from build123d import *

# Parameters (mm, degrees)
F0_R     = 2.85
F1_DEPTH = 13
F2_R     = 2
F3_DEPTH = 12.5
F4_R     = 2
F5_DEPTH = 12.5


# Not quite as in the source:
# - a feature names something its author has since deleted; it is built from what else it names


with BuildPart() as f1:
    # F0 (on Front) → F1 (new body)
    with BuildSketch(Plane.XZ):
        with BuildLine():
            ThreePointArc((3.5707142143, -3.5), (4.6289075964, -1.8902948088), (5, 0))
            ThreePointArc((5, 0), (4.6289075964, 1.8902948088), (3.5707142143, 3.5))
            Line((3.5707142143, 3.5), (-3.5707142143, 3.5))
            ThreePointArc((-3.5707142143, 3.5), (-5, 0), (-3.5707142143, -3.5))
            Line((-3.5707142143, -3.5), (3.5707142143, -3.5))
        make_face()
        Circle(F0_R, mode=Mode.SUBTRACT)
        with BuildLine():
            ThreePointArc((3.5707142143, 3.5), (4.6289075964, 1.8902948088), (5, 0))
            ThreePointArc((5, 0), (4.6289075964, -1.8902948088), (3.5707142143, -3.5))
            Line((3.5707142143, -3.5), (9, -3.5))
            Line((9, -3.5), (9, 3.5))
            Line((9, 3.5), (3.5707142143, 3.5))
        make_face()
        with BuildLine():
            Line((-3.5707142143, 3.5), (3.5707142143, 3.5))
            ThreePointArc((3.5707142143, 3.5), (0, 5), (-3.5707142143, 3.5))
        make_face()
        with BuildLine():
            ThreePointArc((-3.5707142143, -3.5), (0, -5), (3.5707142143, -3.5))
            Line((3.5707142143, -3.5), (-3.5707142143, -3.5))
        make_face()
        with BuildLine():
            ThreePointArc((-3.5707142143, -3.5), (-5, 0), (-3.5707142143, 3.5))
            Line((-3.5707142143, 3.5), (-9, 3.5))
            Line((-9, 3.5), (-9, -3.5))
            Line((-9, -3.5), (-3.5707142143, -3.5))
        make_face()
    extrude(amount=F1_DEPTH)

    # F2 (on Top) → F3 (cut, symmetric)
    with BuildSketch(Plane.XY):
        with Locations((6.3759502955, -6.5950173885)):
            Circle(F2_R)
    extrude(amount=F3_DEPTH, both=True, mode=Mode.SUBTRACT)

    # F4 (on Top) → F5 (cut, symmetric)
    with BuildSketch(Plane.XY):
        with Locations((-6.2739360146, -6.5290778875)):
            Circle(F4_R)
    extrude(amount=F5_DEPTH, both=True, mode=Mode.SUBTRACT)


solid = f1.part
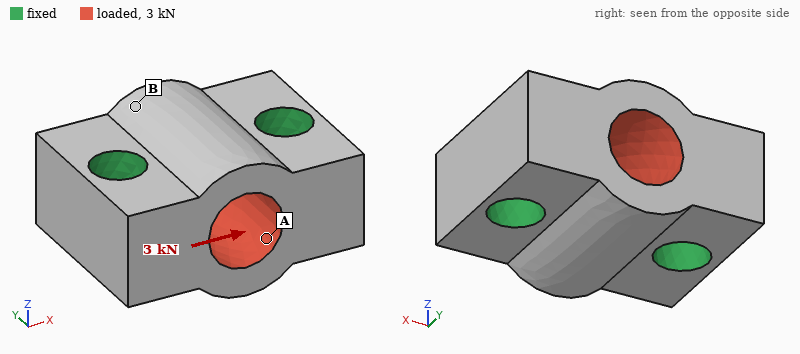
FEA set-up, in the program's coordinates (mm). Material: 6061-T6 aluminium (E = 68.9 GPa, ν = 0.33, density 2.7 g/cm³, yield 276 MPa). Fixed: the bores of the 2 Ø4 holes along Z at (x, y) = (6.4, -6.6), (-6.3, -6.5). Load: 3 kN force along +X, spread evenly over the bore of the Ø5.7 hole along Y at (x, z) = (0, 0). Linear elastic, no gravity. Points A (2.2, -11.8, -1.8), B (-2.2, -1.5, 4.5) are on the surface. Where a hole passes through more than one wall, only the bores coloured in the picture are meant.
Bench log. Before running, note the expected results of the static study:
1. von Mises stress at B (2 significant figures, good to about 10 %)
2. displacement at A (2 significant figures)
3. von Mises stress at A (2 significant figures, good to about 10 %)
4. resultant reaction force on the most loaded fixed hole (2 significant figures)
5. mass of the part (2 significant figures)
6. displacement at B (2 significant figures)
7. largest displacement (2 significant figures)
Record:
8.4 MPa
2.2 µm
20 MPa
1.5 kN
3.6 g
1.9 µm
2.6 µm
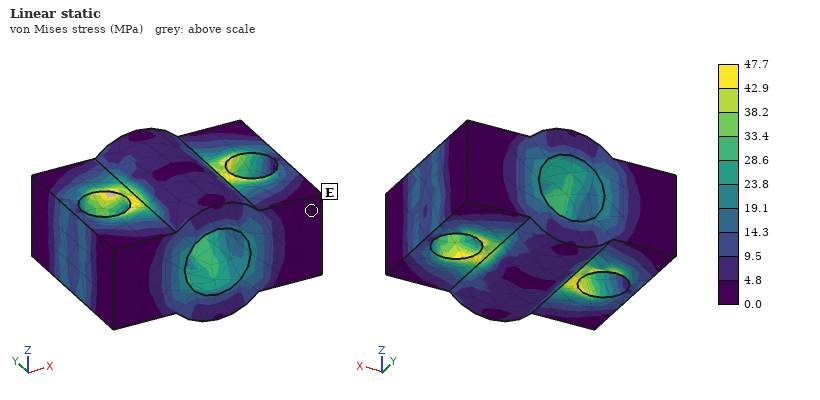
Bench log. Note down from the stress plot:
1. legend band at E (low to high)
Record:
0.0 to 4.8 MPa
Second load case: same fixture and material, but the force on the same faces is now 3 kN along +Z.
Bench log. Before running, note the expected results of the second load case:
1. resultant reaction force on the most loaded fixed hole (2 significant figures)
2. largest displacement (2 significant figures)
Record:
1.5 kN
5.7 µm
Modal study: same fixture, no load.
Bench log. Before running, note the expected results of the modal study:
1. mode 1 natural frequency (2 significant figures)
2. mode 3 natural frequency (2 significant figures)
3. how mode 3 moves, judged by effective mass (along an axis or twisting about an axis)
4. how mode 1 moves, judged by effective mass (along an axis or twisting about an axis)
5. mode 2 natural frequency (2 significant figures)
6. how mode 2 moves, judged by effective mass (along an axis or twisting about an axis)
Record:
87 kHz
100 kHz
along Z
twisting about X
94 kHz
along Y
